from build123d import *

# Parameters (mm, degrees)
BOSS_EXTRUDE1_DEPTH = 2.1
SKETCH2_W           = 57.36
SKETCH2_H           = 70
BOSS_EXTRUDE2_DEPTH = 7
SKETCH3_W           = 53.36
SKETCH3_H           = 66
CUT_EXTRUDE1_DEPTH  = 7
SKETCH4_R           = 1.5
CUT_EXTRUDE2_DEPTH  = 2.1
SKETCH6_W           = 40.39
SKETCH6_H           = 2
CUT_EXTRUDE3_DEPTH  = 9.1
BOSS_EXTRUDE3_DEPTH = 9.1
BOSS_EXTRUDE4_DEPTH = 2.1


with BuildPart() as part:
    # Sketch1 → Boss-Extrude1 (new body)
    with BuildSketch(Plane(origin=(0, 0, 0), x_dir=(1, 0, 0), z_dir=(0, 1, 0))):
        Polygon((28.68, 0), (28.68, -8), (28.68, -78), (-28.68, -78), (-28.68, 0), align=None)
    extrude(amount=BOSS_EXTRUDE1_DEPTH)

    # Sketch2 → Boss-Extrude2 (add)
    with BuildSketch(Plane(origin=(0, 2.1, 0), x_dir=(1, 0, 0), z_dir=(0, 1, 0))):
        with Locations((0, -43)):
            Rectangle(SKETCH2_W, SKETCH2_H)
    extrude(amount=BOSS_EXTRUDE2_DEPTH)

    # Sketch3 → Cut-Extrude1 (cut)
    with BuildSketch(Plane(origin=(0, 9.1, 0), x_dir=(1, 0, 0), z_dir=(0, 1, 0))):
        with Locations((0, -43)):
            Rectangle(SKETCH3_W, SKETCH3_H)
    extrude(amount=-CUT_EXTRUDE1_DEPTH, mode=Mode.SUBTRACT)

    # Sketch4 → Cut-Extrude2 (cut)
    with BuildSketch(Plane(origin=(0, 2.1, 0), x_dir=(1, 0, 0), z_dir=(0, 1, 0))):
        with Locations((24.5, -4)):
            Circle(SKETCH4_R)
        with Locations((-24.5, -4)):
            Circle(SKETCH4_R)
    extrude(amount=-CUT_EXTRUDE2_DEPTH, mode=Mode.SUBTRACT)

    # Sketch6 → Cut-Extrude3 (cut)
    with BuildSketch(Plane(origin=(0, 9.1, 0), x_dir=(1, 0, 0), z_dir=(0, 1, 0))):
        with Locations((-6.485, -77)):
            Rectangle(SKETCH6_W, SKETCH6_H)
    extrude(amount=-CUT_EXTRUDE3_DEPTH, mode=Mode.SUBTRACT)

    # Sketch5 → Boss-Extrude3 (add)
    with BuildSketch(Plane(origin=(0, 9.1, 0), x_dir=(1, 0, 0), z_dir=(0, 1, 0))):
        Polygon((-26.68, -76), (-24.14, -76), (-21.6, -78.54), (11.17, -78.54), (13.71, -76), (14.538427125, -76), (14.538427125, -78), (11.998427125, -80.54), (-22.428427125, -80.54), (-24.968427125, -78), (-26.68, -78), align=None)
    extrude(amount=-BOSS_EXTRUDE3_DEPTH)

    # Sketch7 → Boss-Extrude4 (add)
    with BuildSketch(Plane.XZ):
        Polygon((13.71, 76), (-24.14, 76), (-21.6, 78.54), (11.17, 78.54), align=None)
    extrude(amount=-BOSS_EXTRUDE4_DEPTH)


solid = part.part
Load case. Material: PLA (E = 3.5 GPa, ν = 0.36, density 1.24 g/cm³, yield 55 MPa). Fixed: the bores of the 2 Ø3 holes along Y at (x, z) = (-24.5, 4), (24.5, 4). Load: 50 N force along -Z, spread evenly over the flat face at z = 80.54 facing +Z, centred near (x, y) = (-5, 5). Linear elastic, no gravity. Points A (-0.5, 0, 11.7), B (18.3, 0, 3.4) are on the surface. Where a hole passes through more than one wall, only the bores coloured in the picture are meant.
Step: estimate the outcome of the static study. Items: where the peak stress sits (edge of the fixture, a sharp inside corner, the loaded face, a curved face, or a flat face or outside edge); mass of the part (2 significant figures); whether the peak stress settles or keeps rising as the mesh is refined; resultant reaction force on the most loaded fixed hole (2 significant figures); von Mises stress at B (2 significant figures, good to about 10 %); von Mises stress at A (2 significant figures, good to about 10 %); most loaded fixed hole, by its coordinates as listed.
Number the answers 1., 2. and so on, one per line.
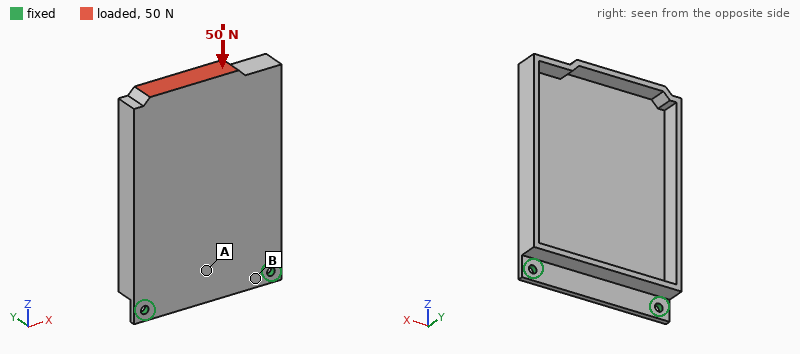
1. edge of the fixture
2. 16 g
3. keeps rising
4. 30 N
5. 3.1 MPa
6. 0.66 MPa
7. (-24.5, 4)
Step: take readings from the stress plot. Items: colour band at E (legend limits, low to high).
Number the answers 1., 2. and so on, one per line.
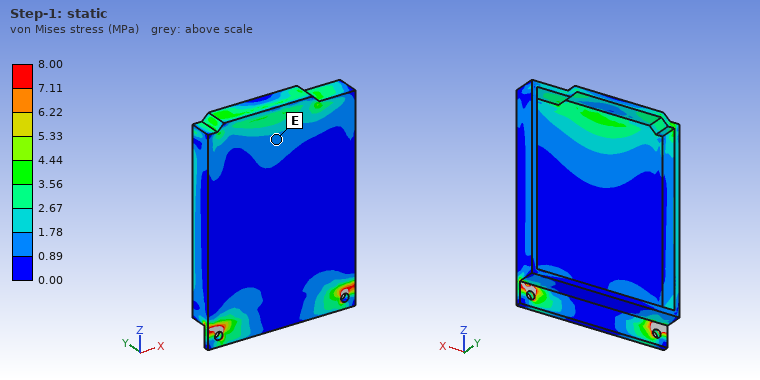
1. 0.89 to 1.78 MPa
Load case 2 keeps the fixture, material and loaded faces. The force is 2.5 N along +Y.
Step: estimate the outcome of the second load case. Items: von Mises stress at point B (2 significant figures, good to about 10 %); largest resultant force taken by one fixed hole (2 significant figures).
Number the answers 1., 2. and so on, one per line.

1. 3.7 MPa
2. 6.1 N
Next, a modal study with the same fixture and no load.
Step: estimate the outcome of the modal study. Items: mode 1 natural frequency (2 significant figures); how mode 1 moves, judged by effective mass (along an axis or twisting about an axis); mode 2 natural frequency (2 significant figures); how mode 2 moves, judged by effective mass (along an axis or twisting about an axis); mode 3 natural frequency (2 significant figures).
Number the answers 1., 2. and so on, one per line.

1. 110 Hz
2. along Y
3. 290 Hz
4. twisting about Z
5. 1000 Hz
